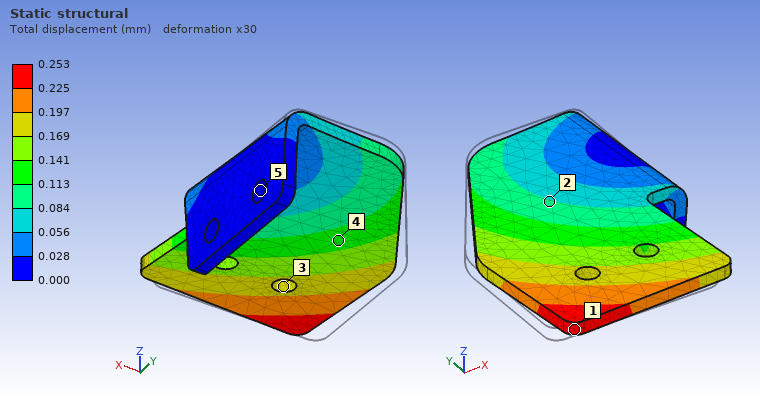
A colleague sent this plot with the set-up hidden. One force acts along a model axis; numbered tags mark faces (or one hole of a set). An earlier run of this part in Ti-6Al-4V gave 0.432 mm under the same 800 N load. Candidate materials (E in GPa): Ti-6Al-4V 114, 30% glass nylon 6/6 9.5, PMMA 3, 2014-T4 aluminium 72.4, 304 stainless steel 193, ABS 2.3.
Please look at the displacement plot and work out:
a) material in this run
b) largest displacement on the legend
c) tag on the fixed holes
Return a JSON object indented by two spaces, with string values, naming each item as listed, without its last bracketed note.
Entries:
{
  "material in this run": "304 stainless steel",
  "largest displacement on the legend": "0.253 mm",
  "tag on the fixed holes": "5"
}
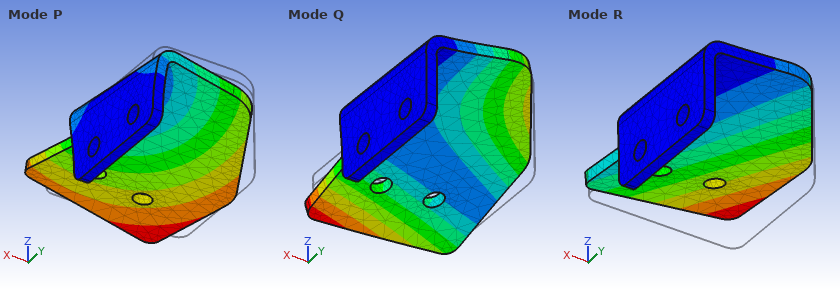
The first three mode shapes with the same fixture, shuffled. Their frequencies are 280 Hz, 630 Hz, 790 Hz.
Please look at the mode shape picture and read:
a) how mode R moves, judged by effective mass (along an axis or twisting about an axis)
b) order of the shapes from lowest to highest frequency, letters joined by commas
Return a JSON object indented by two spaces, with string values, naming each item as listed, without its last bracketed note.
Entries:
{
  "how mode R moves, judged by effective mass": "along Z",
  "order of the shapes from lowest to highest frequency, letters joined by commas": "R, P, Q"
}
